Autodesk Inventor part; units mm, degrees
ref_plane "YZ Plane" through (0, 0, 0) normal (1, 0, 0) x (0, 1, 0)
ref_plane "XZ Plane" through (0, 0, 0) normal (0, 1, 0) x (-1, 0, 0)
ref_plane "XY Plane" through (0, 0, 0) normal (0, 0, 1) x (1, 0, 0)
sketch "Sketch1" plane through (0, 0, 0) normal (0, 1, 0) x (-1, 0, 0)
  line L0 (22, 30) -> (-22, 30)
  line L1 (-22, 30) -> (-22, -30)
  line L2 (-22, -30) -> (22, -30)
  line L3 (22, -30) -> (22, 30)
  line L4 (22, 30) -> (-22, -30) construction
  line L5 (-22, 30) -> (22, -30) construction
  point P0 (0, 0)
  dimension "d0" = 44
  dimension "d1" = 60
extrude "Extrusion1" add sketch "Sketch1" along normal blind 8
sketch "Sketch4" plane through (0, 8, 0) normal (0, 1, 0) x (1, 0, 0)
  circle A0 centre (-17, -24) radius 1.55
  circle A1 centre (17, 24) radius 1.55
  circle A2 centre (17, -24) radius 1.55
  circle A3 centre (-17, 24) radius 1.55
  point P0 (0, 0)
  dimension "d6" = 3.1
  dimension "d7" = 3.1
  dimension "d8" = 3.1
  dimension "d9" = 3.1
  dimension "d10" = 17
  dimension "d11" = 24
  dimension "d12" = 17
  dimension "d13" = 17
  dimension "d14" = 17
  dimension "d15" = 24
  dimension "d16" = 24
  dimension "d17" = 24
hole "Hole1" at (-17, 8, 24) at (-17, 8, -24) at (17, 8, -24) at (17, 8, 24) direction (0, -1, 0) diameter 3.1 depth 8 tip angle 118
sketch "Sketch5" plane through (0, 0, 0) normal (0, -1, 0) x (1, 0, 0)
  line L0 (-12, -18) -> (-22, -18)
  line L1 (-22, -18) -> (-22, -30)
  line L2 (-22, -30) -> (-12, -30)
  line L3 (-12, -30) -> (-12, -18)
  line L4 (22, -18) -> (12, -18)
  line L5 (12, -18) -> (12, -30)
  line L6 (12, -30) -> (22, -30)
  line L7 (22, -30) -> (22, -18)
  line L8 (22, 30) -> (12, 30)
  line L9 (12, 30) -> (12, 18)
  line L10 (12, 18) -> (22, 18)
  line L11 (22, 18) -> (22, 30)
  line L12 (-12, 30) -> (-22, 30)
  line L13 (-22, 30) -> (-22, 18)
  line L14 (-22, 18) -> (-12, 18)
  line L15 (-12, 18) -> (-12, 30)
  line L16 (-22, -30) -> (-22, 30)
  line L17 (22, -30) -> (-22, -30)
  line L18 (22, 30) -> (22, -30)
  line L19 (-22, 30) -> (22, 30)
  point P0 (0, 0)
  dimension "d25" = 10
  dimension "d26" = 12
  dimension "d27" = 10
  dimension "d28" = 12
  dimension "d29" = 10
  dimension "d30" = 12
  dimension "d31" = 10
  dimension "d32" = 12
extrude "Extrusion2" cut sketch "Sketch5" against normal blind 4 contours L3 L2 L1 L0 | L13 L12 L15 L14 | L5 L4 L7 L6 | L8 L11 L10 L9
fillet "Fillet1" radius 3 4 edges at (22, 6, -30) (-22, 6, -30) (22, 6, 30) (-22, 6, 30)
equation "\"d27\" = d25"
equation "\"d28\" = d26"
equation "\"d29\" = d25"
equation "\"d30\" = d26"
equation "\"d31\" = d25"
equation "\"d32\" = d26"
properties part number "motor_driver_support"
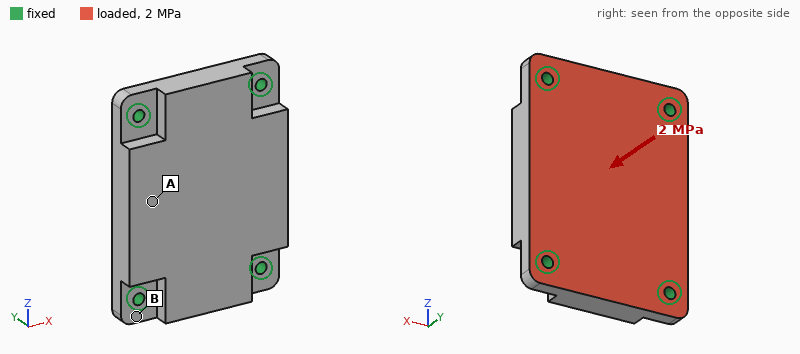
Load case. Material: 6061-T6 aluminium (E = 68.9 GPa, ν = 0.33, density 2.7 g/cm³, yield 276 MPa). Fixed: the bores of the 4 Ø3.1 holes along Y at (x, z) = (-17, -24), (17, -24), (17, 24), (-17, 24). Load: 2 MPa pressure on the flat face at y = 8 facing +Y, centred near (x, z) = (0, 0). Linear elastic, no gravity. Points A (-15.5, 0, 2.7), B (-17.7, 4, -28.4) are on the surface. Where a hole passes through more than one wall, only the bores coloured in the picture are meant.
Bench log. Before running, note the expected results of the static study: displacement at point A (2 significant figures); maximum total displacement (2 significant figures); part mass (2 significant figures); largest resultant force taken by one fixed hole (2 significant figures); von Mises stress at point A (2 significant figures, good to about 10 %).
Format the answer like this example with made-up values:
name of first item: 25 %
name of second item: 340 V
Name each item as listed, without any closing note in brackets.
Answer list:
displacement at point A: 30 µm
maximum total displacement: 32 µm
part mass: 51 g
largest resultant force taken by one fixed hole: 1.5 kN
von Mises stress at point A: 34 MPa
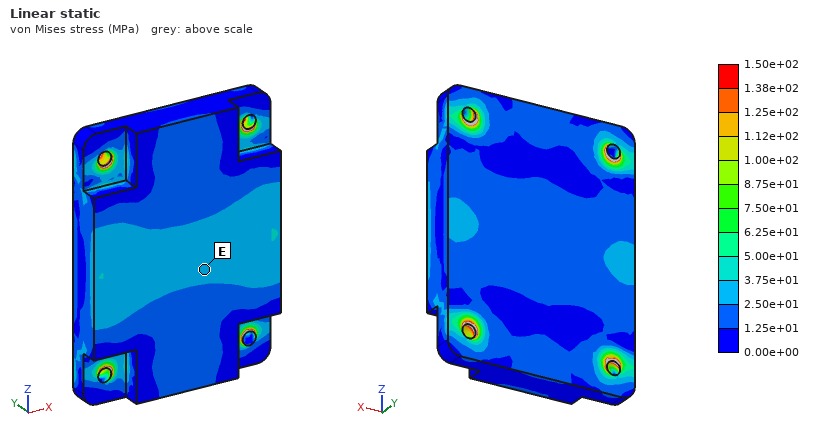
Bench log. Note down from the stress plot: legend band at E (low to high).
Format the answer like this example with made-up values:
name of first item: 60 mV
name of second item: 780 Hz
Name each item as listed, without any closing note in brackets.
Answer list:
legend band at E: 2.50e+01 to 3.75e+01 MPa
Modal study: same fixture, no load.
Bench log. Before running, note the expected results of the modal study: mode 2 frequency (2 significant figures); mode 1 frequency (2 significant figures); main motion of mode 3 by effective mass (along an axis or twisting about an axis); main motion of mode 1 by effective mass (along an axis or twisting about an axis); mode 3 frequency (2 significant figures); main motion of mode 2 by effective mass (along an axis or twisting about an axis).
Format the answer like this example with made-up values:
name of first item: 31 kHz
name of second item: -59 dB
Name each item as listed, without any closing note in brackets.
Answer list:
mode 2 frequency: 14 kHz
mode 1 frequency: 9600 Hz
main motion of mode 3 by effective mass: twisting about X
main motion of mode 1 by effective mass: along Y
mode 3 frequency: 19 kHz
main motion of mode 2 by effective mass: twisting about Z
